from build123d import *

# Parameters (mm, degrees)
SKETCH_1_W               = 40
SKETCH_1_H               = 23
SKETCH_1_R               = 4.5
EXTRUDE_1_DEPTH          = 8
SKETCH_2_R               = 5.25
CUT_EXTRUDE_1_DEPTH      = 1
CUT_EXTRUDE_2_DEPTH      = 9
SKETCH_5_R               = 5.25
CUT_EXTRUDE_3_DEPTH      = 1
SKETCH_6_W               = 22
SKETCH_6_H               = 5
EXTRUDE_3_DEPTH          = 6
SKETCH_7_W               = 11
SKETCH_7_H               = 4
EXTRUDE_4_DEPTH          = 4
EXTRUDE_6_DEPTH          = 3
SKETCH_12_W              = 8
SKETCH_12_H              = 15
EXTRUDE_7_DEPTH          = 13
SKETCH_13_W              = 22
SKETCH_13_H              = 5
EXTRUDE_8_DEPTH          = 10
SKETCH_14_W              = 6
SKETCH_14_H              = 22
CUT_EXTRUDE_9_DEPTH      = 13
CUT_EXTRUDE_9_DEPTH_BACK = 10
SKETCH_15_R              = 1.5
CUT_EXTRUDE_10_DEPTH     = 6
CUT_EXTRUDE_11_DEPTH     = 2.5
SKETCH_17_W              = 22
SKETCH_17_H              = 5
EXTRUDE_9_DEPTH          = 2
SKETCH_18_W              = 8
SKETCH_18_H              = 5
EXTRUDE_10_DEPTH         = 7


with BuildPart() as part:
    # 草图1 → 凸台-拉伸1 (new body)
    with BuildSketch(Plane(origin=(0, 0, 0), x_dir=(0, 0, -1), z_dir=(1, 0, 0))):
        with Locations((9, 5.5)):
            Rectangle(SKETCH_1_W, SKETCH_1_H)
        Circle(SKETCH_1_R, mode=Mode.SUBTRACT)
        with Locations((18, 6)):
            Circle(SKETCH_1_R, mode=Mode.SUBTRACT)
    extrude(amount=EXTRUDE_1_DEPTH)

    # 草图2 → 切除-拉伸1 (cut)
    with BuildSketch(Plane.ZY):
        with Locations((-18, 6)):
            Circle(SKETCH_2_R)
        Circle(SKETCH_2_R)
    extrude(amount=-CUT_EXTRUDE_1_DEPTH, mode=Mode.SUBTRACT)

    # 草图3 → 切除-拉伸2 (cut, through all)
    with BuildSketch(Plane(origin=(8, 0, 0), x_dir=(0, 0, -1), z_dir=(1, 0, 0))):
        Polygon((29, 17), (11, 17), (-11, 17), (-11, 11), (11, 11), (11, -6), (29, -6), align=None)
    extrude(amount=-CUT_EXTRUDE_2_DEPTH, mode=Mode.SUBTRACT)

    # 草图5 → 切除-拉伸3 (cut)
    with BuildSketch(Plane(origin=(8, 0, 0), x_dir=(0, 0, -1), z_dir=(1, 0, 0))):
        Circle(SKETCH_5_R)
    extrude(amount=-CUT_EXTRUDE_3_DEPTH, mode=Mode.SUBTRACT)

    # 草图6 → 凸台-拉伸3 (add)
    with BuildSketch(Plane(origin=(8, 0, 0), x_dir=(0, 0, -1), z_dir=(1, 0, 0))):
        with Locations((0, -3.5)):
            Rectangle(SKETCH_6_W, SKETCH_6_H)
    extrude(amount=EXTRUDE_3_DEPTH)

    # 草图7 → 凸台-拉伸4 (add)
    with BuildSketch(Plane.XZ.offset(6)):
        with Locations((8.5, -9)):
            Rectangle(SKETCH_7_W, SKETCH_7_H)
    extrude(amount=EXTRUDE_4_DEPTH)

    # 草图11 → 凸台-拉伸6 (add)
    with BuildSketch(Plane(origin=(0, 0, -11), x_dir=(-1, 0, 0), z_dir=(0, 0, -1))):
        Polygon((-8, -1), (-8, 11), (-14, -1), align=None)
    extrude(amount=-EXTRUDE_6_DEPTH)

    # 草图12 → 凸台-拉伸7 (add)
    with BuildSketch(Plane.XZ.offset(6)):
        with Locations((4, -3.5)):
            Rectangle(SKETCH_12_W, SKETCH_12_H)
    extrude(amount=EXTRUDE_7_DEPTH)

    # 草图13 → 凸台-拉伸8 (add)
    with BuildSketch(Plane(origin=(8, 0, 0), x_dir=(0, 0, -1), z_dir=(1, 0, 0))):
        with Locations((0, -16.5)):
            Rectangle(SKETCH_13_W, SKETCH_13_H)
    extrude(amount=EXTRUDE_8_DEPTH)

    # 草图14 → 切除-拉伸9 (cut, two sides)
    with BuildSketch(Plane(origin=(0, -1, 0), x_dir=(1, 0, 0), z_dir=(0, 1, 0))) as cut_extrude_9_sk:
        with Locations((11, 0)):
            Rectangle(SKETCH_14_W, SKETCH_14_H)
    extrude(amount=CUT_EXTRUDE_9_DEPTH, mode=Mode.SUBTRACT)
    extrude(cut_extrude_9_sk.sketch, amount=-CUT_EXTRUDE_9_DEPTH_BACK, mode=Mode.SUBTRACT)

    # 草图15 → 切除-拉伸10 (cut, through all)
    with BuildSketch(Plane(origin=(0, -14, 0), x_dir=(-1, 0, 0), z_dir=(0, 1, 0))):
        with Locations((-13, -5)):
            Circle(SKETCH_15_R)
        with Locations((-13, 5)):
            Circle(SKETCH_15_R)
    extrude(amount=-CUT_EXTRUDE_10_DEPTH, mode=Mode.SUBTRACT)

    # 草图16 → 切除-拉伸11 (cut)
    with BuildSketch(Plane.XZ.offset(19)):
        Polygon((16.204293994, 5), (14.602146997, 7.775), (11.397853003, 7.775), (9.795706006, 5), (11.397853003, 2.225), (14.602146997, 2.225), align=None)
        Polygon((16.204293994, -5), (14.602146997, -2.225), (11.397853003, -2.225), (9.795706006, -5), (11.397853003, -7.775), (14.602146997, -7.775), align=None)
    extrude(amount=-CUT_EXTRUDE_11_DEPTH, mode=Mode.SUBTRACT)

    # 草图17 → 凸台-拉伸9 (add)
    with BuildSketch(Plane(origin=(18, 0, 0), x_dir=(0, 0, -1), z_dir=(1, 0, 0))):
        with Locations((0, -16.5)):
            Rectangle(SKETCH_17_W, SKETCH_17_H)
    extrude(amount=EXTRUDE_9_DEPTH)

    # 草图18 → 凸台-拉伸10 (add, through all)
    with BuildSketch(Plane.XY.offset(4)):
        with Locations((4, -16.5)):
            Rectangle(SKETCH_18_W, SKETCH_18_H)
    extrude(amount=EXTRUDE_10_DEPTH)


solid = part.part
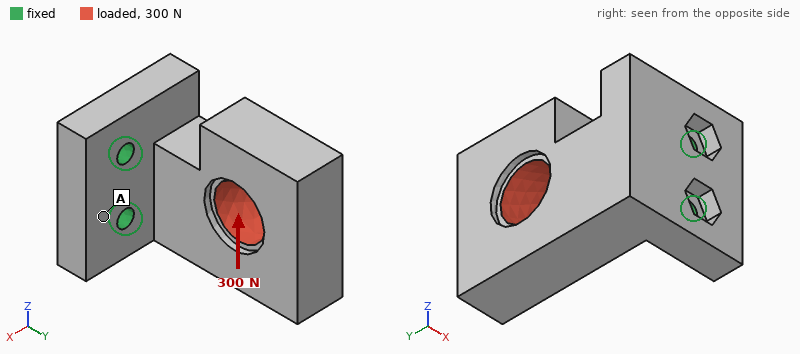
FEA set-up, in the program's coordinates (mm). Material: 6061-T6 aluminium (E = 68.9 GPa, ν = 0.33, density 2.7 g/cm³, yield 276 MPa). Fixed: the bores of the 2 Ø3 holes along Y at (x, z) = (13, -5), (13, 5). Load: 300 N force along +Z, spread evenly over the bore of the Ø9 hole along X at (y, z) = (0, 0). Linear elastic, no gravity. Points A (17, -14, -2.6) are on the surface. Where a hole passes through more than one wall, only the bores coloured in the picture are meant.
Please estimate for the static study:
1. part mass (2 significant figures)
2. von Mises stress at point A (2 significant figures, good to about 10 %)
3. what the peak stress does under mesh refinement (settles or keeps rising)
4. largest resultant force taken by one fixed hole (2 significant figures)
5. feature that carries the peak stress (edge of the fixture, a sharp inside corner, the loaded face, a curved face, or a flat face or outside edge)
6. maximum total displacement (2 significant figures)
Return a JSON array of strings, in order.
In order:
["15 g", "13 MPa", "keeps rising", "460 N", "edge of the fixture", "51 µm"]
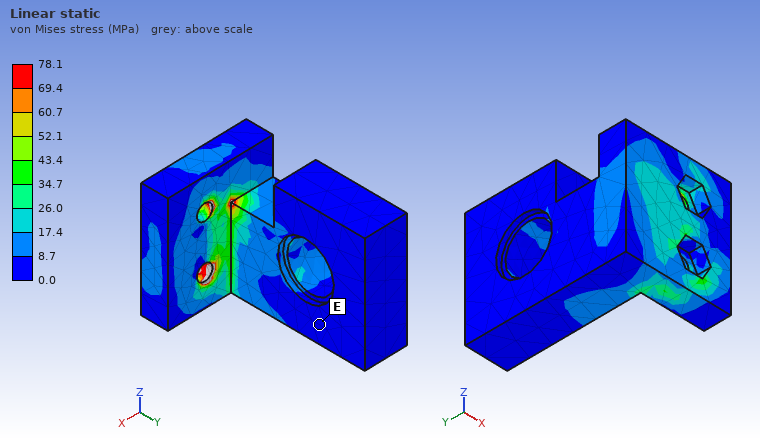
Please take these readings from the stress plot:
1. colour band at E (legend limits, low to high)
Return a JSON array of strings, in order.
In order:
["0.0 to 8.7 MPa"]
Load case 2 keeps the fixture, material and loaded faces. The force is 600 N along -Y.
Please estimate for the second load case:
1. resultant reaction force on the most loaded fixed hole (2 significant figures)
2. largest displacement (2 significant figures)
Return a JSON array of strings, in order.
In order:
["300 N", "0.11 mm"]
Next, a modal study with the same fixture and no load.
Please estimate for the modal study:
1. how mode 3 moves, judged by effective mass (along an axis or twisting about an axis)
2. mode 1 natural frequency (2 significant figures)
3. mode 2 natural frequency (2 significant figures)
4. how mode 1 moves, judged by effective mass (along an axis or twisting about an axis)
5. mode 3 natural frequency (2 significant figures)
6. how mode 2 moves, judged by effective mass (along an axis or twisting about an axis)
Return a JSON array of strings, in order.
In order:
["along Y", "2700 Hz", "4800 Hz", "along X", "11 kHz", "along Z"]
